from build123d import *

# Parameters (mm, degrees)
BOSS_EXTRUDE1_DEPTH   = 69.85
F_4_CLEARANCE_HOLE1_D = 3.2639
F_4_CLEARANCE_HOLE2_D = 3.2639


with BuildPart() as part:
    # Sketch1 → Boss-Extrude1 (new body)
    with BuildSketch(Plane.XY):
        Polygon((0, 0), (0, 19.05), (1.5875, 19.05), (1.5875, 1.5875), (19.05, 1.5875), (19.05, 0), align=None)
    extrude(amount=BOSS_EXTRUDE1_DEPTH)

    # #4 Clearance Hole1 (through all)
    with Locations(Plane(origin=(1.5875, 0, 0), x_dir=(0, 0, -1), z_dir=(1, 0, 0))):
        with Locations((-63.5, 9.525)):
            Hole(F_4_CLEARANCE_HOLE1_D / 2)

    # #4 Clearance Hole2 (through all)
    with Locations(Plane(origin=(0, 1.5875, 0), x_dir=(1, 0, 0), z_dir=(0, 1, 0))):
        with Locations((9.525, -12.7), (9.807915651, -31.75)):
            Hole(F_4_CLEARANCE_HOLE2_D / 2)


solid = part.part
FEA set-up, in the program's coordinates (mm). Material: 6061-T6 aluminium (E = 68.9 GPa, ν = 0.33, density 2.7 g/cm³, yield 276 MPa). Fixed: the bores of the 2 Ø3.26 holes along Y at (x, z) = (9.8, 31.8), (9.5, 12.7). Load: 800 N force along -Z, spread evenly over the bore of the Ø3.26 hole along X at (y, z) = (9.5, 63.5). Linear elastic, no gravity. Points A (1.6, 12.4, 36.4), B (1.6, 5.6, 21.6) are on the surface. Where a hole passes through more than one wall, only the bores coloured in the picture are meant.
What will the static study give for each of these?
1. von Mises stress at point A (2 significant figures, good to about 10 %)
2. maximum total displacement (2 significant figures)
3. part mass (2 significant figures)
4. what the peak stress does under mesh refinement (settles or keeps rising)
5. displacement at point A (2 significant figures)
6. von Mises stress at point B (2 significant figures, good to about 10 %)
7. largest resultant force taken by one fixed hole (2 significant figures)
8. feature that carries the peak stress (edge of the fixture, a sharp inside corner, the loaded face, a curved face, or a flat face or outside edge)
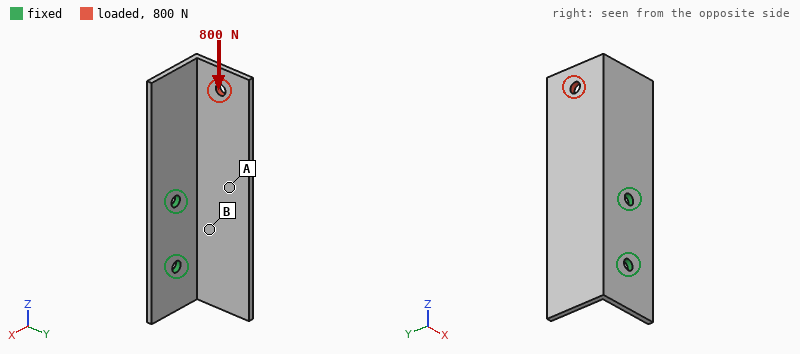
36 MPa
0.51 mm
11 g
keeps rising
0.19 mm
74 MPa
610 N
edge of the fixture
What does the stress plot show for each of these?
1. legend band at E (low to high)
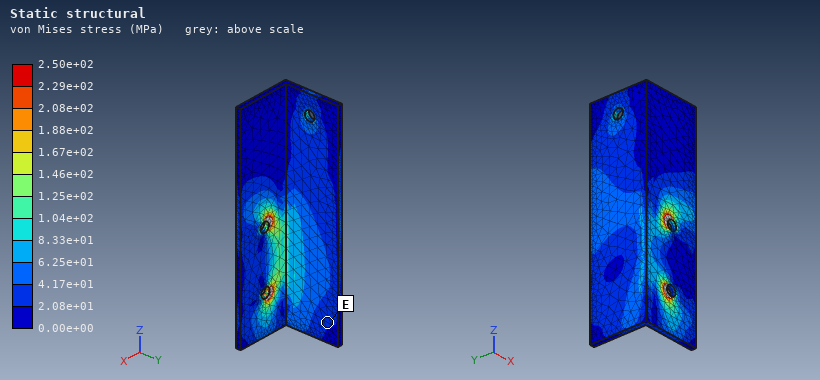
2.08e+01 to 4.17e+01 MPa
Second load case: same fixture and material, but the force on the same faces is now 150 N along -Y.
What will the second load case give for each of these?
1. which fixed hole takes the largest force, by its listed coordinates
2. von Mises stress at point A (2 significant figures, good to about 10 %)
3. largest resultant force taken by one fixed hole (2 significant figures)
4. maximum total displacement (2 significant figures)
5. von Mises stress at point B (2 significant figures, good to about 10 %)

(9.8, 31.8)
25 MPa
340 N
0.57 mm
59 MPa
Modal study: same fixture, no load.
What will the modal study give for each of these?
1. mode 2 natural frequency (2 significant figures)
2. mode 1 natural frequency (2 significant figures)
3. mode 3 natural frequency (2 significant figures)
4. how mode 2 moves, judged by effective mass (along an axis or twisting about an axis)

1900 Hz
1600 Hz
2700 Hz
along Y
